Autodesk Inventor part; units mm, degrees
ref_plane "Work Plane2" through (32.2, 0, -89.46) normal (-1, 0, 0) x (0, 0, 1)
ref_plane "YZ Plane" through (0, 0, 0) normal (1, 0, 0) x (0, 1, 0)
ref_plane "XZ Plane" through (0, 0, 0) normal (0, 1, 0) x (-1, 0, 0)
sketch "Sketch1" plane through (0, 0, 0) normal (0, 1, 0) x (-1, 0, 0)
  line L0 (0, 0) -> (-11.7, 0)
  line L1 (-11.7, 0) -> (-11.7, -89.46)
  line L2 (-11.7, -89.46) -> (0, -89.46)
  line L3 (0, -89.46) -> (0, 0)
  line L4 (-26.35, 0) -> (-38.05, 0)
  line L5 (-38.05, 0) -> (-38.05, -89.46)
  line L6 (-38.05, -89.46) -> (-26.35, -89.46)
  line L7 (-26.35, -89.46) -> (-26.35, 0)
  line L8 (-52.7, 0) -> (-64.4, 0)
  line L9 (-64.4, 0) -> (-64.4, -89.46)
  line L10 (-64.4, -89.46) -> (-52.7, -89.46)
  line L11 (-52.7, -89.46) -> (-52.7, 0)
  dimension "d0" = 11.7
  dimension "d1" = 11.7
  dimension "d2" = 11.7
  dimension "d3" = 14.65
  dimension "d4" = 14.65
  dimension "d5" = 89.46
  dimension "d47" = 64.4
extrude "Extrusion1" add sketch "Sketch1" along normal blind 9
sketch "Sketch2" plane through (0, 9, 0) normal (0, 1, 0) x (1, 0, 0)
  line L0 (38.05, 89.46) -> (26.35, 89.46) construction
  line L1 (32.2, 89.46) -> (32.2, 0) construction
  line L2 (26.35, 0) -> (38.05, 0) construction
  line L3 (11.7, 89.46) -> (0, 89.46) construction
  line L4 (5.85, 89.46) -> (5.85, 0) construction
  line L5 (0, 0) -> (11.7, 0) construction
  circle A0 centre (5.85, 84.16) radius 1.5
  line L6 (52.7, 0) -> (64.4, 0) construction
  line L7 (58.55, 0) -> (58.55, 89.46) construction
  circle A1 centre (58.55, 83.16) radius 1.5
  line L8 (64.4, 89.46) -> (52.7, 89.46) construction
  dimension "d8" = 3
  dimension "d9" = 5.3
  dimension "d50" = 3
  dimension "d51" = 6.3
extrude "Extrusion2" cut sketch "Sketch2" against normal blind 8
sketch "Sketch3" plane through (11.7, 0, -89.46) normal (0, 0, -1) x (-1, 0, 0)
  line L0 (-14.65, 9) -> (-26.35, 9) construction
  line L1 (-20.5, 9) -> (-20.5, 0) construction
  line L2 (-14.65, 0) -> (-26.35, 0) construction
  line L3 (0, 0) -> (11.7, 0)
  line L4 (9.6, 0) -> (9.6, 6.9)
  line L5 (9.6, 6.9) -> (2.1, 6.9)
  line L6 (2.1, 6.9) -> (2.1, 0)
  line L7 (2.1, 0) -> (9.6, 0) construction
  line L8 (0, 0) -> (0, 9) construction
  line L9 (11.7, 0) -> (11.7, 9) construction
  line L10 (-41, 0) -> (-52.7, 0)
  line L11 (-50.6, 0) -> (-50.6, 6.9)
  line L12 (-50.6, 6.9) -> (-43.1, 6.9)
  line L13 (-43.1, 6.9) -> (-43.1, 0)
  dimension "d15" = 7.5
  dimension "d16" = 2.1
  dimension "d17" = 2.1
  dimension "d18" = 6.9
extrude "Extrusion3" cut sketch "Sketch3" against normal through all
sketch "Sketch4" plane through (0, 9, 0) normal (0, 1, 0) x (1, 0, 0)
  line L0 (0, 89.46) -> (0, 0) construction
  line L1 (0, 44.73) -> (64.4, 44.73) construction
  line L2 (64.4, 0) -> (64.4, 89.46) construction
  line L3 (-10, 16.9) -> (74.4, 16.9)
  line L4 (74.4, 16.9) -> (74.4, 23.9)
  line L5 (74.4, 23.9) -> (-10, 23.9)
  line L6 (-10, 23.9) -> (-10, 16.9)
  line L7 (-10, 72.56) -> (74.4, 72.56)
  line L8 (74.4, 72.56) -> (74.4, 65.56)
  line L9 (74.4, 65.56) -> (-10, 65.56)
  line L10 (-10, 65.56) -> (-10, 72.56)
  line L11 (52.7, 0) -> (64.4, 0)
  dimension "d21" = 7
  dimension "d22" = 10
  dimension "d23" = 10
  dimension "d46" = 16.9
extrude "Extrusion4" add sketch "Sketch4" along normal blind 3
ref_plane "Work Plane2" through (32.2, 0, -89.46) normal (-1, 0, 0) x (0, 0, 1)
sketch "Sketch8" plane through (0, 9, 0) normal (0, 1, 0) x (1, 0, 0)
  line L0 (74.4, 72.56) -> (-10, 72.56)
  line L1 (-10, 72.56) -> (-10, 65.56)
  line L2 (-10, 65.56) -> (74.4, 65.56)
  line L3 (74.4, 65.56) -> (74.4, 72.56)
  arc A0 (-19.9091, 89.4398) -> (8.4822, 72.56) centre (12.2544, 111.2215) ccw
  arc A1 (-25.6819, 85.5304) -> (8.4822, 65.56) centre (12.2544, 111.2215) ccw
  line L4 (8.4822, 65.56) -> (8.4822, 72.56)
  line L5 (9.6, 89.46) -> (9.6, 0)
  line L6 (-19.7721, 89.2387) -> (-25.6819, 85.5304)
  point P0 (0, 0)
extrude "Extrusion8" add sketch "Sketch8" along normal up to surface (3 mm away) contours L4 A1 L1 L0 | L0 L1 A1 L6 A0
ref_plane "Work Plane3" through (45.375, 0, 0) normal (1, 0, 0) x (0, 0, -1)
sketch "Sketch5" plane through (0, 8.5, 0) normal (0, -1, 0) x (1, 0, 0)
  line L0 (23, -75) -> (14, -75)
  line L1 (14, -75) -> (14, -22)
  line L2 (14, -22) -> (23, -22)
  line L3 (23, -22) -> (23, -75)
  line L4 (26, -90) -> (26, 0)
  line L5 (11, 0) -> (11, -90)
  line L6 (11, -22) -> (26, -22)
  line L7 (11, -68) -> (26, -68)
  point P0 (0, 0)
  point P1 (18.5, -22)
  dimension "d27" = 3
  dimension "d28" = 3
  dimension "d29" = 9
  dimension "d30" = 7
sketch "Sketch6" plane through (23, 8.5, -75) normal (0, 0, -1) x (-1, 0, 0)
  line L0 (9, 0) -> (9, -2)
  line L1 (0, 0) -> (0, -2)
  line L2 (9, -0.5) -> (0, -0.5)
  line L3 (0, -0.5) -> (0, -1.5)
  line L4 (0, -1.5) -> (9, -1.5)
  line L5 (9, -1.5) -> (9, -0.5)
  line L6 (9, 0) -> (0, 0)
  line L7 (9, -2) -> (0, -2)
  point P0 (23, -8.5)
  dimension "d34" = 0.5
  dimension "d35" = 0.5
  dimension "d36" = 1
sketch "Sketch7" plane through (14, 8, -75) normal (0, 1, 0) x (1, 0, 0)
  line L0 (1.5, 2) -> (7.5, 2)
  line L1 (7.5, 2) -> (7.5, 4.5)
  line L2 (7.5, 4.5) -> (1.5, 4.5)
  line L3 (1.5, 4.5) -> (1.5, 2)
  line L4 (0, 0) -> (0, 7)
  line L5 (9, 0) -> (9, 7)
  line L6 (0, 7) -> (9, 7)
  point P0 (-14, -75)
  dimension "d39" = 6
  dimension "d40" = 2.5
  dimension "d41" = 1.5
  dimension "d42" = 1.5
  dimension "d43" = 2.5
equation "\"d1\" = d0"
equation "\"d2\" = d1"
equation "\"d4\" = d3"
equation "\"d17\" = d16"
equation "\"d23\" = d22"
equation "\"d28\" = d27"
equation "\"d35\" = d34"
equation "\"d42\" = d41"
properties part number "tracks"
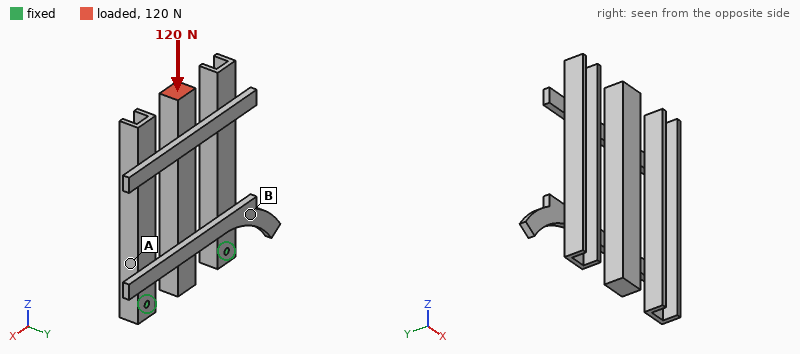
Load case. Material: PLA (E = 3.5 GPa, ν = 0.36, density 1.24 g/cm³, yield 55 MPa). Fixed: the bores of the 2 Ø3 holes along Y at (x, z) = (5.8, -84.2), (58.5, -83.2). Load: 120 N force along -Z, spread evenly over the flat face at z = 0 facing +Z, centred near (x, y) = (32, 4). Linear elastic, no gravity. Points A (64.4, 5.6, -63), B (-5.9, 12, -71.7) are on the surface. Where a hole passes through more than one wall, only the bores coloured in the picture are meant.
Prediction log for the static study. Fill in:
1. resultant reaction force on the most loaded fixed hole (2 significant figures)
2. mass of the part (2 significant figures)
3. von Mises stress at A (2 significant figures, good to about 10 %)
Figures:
61 N
29 g
2.3 MPa
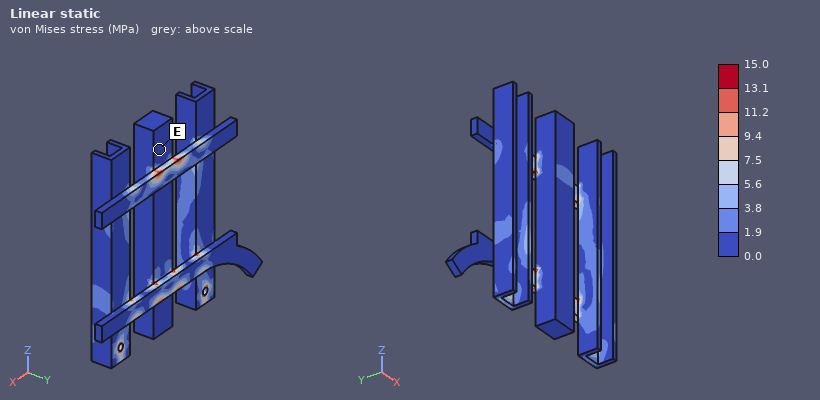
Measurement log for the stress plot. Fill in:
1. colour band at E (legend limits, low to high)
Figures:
0.0 to 1.9 MPa
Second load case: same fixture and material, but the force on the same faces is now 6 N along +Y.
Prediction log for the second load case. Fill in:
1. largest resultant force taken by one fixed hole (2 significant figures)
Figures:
3.0 N
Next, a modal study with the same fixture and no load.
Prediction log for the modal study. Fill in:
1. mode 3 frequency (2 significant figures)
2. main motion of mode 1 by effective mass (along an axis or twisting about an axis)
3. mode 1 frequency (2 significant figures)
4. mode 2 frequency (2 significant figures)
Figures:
500 Hz
along Y
130 Hz
300 Hz
